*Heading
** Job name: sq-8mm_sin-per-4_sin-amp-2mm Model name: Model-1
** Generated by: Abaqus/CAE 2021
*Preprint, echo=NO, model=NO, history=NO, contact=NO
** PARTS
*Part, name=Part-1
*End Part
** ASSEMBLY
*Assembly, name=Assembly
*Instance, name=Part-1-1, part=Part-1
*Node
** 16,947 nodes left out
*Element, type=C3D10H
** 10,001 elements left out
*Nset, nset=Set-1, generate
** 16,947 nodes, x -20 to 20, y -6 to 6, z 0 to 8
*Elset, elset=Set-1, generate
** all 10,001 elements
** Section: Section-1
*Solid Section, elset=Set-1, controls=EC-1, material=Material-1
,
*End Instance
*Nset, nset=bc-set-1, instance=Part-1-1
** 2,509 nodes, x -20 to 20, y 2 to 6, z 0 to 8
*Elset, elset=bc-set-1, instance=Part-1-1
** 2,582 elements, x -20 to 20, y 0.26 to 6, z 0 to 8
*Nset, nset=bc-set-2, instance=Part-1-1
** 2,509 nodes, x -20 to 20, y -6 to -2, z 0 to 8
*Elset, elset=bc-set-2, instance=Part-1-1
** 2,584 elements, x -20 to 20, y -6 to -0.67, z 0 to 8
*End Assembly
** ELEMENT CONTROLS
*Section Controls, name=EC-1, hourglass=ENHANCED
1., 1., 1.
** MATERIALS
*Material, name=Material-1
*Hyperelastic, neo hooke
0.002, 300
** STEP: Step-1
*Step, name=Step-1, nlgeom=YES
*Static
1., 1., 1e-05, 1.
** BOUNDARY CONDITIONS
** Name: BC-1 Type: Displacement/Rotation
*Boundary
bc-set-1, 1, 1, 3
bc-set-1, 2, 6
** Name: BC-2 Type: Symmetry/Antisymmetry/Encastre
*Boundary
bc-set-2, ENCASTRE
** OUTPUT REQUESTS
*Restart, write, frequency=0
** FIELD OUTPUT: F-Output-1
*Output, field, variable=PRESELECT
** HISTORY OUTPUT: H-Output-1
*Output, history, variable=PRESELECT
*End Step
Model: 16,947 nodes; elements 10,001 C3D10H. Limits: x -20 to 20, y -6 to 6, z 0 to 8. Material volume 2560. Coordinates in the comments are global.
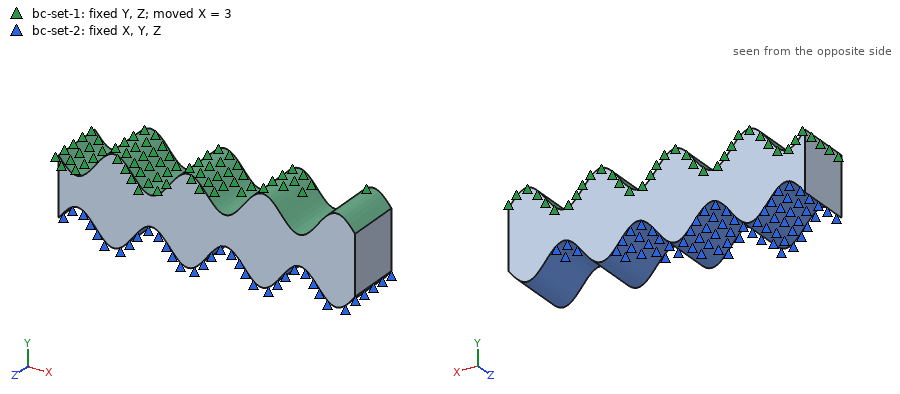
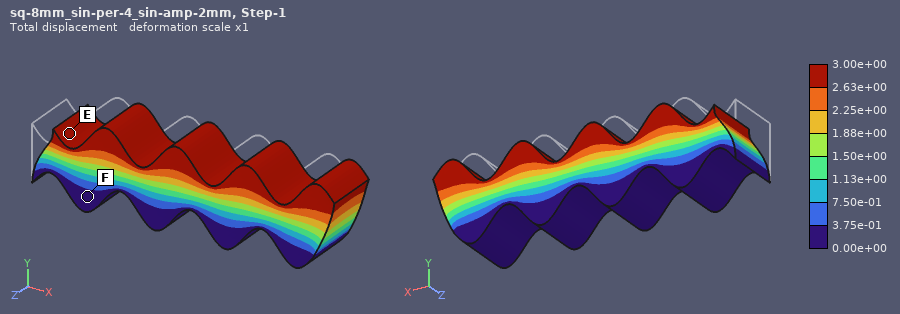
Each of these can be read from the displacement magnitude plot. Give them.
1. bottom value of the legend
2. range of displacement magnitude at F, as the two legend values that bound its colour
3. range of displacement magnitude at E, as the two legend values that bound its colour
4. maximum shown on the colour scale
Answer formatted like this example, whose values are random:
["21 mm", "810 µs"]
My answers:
["0.00e+00", "0.00e+00 to 3.75e-01", "2.63e+00 to 3.00e+00", "3.00e+00"]
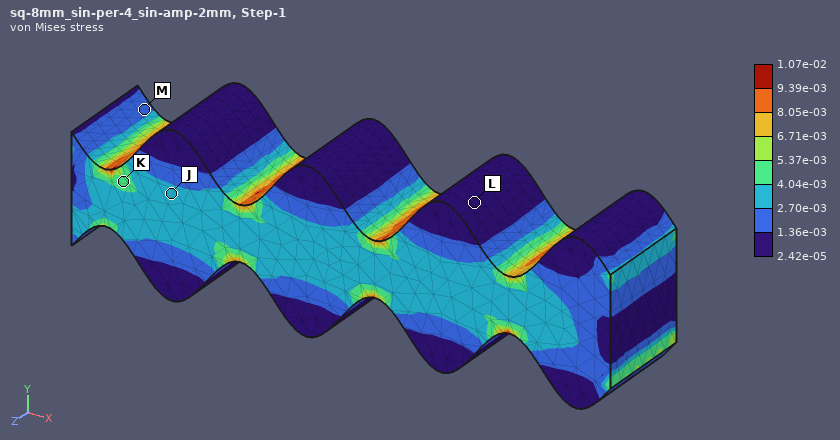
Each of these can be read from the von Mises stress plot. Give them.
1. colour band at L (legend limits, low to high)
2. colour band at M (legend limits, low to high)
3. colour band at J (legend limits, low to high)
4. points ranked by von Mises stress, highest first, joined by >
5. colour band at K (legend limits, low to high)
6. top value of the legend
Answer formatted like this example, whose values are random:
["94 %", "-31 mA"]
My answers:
["2.42e-05 to 1.36e-03", "1.36e-03 to 2.70e-03", "2.70e-03 to 4.04e-03", "K > J > M > L", "4.04e-03 to 5.37e-03", "1.07e-02"]
